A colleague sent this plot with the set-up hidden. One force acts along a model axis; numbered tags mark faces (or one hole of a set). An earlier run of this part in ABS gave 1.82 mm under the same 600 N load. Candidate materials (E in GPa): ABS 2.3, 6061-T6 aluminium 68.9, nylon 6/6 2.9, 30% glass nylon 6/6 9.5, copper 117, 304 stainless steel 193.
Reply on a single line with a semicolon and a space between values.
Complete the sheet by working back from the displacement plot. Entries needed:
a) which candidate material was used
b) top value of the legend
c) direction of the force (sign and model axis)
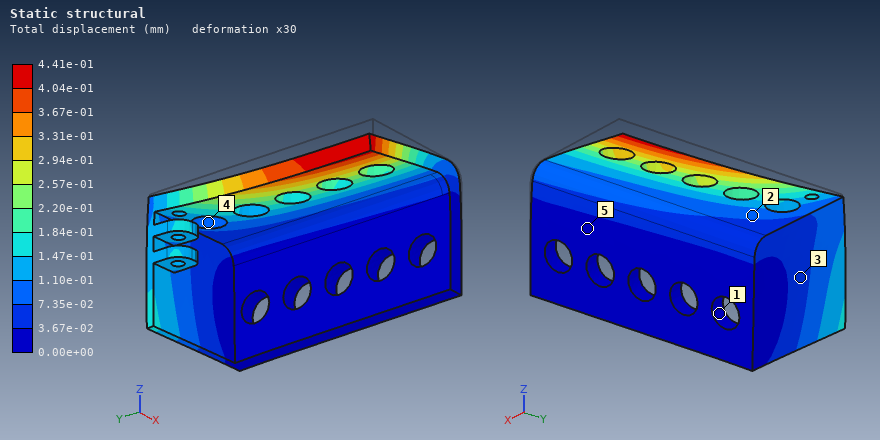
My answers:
30% glass nylon 6/6; 4.41e-01 mm; -Z
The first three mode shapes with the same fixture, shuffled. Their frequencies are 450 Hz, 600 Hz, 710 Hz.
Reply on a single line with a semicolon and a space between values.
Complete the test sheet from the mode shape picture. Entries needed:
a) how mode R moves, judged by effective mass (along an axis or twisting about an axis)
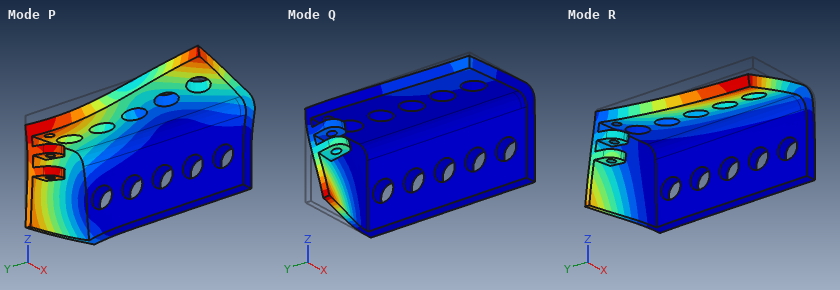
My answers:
along Z
